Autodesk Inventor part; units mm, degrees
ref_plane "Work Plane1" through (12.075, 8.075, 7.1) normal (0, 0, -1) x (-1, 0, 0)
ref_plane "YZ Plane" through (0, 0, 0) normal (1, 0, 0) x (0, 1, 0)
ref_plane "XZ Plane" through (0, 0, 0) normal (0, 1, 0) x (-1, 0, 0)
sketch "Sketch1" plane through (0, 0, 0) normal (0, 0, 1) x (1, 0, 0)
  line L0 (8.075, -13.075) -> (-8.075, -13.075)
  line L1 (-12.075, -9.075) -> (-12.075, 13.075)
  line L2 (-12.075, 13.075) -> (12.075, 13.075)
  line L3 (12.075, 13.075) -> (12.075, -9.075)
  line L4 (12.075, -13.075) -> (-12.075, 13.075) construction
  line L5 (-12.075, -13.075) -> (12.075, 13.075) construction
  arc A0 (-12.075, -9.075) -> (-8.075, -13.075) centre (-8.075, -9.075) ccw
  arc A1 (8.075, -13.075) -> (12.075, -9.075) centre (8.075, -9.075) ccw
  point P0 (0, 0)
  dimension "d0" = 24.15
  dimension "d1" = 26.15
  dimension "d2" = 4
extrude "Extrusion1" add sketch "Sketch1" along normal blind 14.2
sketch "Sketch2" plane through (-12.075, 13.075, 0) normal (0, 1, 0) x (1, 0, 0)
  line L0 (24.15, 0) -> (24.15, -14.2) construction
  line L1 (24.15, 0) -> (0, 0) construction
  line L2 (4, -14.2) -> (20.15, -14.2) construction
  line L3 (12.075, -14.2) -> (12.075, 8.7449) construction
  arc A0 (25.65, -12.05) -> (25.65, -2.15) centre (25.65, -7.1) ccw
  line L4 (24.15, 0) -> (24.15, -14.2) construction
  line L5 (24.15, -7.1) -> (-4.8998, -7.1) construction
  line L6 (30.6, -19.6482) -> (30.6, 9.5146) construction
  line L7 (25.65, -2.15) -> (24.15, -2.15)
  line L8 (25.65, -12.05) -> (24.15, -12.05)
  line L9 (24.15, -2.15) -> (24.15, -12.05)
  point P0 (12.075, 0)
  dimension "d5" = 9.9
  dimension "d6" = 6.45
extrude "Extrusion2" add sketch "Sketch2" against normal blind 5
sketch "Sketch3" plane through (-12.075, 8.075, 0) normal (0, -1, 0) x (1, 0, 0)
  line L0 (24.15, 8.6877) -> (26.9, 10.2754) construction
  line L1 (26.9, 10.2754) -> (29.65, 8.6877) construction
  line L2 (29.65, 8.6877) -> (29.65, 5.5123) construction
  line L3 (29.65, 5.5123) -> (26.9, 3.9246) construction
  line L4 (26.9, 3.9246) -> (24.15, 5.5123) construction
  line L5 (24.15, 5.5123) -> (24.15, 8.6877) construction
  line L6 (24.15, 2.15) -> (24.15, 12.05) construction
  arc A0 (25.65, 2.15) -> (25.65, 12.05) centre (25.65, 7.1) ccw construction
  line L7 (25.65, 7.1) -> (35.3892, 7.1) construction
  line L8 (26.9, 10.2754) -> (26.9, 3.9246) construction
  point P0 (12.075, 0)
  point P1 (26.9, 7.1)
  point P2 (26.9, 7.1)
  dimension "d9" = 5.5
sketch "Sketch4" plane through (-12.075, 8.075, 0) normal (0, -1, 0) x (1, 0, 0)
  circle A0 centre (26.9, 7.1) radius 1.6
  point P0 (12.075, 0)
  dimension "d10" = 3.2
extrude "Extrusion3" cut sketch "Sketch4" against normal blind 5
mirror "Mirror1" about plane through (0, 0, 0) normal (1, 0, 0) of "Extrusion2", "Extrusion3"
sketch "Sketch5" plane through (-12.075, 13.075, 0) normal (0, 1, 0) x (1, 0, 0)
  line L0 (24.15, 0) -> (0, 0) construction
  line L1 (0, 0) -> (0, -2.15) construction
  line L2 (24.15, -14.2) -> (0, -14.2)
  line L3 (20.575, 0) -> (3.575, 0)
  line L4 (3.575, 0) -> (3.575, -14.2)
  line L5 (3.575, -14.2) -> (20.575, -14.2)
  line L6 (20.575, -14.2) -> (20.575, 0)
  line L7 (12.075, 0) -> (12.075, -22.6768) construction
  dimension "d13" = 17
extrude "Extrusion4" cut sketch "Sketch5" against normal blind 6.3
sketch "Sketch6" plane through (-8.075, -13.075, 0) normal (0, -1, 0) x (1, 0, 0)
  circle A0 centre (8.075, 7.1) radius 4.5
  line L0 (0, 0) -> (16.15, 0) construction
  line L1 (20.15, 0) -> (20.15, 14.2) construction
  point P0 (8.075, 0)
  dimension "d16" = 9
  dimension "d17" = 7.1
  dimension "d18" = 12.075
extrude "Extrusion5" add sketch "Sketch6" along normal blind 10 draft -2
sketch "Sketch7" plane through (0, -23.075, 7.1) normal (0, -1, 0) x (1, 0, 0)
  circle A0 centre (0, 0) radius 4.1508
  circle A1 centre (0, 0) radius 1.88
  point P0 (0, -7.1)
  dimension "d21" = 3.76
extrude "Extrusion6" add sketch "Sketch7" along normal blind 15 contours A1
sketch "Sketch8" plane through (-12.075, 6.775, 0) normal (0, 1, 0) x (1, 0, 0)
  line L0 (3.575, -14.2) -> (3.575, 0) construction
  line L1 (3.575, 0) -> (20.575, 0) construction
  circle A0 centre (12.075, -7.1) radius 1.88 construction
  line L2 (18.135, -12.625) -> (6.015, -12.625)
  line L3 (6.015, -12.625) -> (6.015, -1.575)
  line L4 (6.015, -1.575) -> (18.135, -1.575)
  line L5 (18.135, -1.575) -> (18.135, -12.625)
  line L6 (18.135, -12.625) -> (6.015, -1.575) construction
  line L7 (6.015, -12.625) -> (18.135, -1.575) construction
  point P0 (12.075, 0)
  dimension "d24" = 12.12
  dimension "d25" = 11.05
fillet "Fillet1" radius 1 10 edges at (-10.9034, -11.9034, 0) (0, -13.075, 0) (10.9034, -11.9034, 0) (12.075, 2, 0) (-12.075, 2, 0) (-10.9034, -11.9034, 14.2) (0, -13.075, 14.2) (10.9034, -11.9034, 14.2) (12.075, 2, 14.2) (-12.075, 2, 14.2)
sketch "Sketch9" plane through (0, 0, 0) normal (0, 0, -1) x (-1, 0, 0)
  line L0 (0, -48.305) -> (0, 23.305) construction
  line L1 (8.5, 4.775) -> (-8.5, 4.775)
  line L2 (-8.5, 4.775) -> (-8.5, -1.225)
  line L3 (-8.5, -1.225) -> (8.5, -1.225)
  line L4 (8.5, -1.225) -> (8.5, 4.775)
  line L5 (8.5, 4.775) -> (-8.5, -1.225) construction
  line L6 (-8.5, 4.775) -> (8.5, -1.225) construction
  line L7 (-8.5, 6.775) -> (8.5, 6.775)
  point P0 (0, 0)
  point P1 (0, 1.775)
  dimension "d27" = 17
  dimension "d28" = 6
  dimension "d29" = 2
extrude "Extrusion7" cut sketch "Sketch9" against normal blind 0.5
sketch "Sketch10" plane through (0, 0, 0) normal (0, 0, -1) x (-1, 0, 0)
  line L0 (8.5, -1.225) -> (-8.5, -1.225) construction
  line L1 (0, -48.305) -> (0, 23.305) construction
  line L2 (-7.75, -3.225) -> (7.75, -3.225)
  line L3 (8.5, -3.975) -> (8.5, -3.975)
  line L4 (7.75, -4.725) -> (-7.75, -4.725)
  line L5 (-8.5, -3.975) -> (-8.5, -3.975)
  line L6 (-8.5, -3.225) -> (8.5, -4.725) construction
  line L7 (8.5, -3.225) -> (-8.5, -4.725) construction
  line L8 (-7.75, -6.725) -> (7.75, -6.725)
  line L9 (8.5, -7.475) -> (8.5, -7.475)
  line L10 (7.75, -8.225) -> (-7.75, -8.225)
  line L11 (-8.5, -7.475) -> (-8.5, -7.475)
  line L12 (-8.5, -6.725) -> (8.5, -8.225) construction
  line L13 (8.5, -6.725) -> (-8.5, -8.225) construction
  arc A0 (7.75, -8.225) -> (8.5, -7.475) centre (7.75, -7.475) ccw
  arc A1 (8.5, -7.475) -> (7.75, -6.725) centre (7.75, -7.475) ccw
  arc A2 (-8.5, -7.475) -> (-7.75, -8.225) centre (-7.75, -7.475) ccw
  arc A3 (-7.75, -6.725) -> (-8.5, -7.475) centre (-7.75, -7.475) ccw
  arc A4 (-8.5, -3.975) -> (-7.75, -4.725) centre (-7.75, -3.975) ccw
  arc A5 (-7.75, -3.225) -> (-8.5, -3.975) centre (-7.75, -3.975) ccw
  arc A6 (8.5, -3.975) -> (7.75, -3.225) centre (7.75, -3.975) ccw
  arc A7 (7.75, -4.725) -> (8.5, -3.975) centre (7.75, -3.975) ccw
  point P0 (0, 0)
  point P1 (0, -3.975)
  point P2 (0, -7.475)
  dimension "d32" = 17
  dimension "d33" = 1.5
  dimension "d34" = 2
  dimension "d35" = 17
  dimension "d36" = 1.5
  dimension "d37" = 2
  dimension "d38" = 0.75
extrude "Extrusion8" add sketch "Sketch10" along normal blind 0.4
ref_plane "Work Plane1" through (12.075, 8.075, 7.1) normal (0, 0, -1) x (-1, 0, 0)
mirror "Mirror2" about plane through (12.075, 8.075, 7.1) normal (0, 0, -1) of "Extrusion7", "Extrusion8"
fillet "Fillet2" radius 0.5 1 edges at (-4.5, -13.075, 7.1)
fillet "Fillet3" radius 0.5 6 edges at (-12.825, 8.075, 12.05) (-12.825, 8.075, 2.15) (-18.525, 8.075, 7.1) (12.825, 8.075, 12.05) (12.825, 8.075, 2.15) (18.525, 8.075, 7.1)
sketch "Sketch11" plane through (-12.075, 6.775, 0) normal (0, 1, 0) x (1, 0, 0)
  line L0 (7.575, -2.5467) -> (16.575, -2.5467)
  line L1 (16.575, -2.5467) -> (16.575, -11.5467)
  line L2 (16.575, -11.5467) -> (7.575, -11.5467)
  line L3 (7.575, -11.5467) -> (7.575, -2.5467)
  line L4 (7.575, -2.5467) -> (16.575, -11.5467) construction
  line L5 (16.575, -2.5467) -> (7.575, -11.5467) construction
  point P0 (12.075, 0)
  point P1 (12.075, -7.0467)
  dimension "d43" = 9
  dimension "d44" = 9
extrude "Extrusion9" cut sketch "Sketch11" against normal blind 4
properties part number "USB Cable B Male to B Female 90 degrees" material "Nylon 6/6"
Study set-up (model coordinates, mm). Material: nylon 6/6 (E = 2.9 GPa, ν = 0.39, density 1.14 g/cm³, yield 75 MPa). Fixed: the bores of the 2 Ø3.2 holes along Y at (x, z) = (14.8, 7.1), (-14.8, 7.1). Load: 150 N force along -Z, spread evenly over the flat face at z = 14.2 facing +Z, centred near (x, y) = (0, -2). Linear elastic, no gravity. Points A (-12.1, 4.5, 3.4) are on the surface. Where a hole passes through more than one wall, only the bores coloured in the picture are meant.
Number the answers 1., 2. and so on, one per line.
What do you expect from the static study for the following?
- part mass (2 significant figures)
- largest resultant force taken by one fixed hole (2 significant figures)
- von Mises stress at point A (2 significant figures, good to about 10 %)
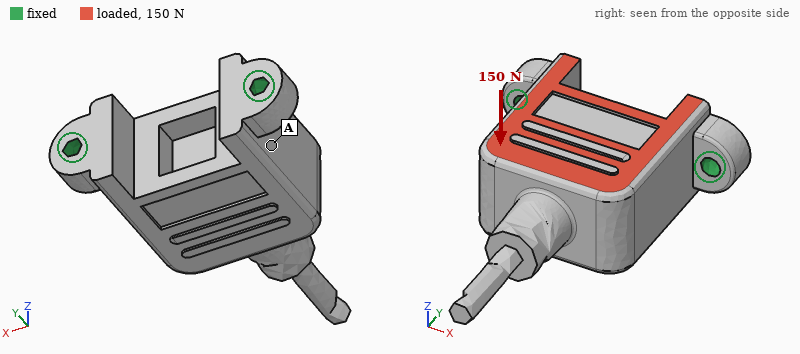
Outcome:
1. 9.3 g
2. 75 N
3. 4.2 MPa
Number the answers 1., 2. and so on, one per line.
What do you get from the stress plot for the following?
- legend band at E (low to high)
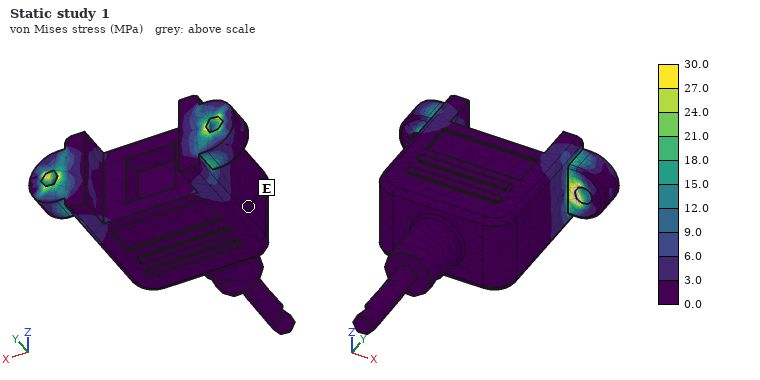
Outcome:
1. 0.0 to 3.0 MPa
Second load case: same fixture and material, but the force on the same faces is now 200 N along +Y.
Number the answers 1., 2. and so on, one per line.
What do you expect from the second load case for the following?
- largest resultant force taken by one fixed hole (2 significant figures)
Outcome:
1. 110 N
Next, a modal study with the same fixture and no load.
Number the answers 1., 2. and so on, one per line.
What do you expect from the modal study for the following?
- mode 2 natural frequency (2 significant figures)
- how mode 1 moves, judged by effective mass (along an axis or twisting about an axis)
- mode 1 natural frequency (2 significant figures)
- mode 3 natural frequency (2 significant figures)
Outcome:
1. 3000 Hz
2. along Z
3. 1200 Hz
4. 3300 Hz
